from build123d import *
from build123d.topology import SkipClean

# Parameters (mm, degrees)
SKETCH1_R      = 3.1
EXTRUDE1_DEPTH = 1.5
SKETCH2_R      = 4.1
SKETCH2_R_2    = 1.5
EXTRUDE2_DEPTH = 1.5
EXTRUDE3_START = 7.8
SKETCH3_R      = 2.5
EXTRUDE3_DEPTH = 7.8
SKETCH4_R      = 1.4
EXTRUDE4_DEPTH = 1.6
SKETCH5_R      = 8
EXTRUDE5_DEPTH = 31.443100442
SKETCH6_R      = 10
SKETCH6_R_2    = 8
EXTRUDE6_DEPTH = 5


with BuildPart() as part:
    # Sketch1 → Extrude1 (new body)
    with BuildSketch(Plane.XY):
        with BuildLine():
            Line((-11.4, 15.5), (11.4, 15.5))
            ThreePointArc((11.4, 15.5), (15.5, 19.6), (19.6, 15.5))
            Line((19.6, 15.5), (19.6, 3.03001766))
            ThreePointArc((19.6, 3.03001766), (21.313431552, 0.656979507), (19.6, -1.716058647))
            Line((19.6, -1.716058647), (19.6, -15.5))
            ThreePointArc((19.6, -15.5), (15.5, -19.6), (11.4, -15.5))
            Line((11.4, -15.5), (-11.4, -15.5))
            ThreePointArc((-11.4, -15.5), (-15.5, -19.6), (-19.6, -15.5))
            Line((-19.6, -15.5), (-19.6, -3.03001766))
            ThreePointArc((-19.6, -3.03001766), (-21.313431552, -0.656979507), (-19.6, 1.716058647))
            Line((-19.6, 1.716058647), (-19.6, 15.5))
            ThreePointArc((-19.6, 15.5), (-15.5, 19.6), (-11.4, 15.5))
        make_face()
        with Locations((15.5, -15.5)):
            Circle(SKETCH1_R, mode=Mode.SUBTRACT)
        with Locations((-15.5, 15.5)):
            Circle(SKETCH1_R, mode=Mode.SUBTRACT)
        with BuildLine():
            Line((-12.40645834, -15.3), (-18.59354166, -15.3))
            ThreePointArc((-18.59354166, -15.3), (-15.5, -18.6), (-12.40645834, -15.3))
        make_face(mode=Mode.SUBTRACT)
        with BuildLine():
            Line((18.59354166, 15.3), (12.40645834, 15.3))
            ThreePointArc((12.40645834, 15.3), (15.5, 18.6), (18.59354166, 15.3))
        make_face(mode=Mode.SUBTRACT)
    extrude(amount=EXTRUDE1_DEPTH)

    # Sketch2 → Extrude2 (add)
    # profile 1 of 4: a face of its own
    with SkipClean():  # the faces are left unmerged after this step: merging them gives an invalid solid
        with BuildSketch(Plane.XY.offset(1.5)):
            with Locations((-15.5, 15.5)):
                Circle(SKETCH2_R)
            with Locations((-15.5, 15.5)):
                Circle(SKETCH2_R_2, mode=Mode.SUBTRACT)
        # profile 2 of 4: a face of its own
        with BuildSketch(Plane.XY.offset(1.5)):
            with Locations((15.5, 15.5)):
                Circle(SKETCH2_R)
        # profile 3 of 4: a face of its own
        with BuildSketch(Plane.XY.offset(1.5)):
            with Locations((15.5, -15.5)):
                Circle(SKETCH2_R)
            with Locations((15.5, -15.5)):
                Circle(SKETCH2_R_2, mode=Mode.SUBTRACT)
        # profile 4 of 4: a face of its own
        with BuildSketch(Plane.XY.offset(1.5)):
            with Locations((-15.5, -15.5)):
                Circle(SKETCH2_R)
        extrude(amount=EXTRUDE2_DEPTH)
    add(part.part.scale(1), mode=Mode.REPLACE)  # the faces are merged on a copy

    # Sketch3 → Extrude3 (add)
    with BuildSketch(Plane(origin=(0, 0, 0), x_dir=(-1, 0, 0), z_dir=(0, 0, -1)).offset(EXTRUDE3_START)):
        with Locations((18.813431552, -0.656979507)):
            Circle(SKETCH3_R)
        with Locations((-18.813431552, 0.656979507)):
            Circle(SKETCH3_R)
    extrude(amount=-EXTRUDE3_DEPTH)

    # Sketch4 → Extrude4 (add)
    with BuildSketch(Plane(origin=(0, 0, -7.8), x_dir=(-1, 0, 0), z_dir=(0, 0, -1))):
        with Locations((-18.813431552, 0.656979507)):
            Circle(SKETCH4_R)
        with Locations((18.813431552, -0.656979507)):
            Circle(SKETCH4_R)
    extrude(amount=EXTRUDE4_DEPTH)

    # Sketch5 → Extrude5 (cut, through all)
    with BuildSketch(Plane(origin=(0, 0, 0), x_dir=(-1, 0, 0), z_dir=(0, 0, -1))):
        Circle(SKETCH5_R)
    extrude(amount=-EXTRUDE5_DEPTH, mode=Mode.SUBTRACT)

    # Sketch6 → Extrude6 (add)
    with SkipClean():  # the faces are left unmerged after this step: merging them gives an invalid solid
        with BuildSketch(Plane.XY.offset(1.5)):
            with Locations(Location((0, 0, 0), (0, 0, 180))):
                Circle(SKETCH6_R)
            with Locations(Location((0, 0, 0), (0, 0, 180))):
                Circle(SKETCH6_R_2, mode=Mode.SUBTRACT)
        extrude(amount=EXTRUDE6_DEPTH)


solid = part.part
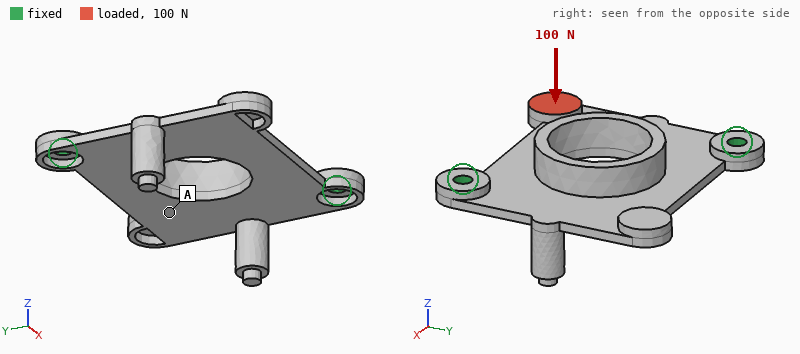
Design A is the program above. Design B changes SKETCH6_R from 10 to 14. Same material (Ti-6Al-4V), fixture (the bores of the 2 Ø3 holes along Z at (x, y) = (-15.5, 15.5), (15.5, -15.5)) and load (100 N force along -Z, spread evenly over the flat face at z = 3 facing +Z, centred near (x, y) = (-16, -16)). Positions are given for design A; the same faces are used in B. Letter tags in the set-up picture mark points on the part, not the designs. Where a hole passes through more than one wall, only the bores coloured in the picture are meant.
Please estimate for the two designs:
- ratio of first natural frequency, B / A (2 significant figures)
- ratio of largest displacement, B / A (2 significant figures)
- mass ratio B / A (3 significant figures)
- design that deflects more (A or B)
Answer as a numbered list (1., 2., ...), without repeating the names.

1. 1.1
2. 0.55
3. 1.55
4. A
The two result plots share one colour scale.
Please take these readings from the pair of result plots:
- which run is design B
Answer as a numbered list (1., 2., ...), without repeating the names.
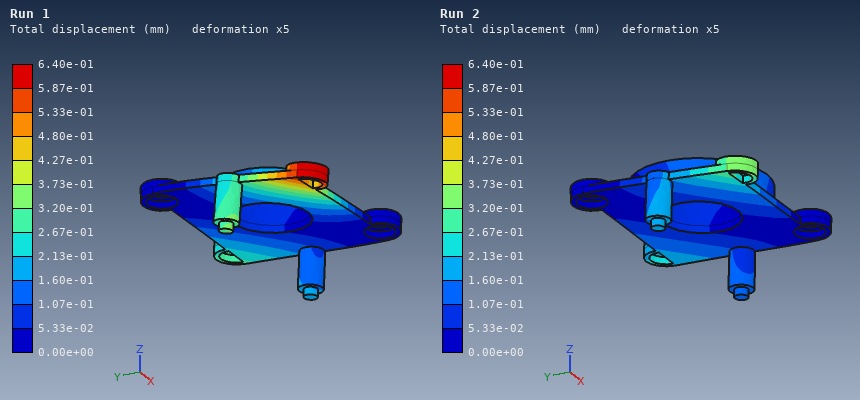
1. Run 2
